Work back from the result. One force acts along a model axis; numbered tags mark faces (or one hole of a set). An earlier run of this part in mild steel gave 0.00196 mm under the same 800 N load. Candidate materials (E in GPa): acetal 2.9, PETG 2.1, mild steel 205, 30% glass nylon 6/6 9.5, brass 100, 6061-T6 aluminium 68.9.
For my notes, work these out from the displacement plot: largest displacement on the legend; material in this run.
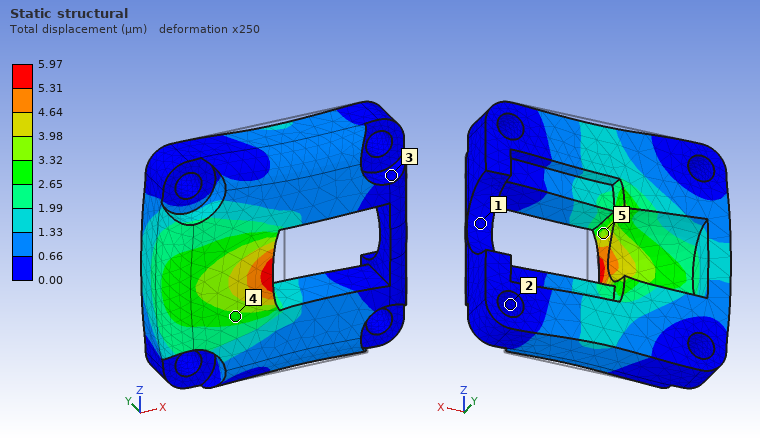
5.97 µm
6061-T6 aluminium
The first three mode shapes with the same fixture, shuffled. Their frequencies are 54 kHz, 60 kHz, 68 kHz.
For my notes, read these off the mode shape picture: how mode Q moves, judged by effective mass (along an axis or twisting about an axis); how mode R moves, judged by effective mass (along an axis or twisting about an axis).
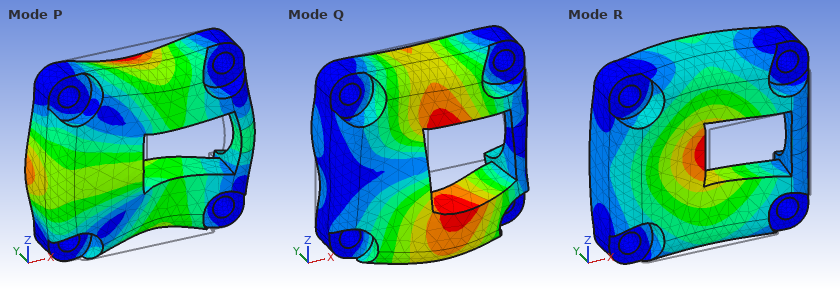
along Z
along Y
